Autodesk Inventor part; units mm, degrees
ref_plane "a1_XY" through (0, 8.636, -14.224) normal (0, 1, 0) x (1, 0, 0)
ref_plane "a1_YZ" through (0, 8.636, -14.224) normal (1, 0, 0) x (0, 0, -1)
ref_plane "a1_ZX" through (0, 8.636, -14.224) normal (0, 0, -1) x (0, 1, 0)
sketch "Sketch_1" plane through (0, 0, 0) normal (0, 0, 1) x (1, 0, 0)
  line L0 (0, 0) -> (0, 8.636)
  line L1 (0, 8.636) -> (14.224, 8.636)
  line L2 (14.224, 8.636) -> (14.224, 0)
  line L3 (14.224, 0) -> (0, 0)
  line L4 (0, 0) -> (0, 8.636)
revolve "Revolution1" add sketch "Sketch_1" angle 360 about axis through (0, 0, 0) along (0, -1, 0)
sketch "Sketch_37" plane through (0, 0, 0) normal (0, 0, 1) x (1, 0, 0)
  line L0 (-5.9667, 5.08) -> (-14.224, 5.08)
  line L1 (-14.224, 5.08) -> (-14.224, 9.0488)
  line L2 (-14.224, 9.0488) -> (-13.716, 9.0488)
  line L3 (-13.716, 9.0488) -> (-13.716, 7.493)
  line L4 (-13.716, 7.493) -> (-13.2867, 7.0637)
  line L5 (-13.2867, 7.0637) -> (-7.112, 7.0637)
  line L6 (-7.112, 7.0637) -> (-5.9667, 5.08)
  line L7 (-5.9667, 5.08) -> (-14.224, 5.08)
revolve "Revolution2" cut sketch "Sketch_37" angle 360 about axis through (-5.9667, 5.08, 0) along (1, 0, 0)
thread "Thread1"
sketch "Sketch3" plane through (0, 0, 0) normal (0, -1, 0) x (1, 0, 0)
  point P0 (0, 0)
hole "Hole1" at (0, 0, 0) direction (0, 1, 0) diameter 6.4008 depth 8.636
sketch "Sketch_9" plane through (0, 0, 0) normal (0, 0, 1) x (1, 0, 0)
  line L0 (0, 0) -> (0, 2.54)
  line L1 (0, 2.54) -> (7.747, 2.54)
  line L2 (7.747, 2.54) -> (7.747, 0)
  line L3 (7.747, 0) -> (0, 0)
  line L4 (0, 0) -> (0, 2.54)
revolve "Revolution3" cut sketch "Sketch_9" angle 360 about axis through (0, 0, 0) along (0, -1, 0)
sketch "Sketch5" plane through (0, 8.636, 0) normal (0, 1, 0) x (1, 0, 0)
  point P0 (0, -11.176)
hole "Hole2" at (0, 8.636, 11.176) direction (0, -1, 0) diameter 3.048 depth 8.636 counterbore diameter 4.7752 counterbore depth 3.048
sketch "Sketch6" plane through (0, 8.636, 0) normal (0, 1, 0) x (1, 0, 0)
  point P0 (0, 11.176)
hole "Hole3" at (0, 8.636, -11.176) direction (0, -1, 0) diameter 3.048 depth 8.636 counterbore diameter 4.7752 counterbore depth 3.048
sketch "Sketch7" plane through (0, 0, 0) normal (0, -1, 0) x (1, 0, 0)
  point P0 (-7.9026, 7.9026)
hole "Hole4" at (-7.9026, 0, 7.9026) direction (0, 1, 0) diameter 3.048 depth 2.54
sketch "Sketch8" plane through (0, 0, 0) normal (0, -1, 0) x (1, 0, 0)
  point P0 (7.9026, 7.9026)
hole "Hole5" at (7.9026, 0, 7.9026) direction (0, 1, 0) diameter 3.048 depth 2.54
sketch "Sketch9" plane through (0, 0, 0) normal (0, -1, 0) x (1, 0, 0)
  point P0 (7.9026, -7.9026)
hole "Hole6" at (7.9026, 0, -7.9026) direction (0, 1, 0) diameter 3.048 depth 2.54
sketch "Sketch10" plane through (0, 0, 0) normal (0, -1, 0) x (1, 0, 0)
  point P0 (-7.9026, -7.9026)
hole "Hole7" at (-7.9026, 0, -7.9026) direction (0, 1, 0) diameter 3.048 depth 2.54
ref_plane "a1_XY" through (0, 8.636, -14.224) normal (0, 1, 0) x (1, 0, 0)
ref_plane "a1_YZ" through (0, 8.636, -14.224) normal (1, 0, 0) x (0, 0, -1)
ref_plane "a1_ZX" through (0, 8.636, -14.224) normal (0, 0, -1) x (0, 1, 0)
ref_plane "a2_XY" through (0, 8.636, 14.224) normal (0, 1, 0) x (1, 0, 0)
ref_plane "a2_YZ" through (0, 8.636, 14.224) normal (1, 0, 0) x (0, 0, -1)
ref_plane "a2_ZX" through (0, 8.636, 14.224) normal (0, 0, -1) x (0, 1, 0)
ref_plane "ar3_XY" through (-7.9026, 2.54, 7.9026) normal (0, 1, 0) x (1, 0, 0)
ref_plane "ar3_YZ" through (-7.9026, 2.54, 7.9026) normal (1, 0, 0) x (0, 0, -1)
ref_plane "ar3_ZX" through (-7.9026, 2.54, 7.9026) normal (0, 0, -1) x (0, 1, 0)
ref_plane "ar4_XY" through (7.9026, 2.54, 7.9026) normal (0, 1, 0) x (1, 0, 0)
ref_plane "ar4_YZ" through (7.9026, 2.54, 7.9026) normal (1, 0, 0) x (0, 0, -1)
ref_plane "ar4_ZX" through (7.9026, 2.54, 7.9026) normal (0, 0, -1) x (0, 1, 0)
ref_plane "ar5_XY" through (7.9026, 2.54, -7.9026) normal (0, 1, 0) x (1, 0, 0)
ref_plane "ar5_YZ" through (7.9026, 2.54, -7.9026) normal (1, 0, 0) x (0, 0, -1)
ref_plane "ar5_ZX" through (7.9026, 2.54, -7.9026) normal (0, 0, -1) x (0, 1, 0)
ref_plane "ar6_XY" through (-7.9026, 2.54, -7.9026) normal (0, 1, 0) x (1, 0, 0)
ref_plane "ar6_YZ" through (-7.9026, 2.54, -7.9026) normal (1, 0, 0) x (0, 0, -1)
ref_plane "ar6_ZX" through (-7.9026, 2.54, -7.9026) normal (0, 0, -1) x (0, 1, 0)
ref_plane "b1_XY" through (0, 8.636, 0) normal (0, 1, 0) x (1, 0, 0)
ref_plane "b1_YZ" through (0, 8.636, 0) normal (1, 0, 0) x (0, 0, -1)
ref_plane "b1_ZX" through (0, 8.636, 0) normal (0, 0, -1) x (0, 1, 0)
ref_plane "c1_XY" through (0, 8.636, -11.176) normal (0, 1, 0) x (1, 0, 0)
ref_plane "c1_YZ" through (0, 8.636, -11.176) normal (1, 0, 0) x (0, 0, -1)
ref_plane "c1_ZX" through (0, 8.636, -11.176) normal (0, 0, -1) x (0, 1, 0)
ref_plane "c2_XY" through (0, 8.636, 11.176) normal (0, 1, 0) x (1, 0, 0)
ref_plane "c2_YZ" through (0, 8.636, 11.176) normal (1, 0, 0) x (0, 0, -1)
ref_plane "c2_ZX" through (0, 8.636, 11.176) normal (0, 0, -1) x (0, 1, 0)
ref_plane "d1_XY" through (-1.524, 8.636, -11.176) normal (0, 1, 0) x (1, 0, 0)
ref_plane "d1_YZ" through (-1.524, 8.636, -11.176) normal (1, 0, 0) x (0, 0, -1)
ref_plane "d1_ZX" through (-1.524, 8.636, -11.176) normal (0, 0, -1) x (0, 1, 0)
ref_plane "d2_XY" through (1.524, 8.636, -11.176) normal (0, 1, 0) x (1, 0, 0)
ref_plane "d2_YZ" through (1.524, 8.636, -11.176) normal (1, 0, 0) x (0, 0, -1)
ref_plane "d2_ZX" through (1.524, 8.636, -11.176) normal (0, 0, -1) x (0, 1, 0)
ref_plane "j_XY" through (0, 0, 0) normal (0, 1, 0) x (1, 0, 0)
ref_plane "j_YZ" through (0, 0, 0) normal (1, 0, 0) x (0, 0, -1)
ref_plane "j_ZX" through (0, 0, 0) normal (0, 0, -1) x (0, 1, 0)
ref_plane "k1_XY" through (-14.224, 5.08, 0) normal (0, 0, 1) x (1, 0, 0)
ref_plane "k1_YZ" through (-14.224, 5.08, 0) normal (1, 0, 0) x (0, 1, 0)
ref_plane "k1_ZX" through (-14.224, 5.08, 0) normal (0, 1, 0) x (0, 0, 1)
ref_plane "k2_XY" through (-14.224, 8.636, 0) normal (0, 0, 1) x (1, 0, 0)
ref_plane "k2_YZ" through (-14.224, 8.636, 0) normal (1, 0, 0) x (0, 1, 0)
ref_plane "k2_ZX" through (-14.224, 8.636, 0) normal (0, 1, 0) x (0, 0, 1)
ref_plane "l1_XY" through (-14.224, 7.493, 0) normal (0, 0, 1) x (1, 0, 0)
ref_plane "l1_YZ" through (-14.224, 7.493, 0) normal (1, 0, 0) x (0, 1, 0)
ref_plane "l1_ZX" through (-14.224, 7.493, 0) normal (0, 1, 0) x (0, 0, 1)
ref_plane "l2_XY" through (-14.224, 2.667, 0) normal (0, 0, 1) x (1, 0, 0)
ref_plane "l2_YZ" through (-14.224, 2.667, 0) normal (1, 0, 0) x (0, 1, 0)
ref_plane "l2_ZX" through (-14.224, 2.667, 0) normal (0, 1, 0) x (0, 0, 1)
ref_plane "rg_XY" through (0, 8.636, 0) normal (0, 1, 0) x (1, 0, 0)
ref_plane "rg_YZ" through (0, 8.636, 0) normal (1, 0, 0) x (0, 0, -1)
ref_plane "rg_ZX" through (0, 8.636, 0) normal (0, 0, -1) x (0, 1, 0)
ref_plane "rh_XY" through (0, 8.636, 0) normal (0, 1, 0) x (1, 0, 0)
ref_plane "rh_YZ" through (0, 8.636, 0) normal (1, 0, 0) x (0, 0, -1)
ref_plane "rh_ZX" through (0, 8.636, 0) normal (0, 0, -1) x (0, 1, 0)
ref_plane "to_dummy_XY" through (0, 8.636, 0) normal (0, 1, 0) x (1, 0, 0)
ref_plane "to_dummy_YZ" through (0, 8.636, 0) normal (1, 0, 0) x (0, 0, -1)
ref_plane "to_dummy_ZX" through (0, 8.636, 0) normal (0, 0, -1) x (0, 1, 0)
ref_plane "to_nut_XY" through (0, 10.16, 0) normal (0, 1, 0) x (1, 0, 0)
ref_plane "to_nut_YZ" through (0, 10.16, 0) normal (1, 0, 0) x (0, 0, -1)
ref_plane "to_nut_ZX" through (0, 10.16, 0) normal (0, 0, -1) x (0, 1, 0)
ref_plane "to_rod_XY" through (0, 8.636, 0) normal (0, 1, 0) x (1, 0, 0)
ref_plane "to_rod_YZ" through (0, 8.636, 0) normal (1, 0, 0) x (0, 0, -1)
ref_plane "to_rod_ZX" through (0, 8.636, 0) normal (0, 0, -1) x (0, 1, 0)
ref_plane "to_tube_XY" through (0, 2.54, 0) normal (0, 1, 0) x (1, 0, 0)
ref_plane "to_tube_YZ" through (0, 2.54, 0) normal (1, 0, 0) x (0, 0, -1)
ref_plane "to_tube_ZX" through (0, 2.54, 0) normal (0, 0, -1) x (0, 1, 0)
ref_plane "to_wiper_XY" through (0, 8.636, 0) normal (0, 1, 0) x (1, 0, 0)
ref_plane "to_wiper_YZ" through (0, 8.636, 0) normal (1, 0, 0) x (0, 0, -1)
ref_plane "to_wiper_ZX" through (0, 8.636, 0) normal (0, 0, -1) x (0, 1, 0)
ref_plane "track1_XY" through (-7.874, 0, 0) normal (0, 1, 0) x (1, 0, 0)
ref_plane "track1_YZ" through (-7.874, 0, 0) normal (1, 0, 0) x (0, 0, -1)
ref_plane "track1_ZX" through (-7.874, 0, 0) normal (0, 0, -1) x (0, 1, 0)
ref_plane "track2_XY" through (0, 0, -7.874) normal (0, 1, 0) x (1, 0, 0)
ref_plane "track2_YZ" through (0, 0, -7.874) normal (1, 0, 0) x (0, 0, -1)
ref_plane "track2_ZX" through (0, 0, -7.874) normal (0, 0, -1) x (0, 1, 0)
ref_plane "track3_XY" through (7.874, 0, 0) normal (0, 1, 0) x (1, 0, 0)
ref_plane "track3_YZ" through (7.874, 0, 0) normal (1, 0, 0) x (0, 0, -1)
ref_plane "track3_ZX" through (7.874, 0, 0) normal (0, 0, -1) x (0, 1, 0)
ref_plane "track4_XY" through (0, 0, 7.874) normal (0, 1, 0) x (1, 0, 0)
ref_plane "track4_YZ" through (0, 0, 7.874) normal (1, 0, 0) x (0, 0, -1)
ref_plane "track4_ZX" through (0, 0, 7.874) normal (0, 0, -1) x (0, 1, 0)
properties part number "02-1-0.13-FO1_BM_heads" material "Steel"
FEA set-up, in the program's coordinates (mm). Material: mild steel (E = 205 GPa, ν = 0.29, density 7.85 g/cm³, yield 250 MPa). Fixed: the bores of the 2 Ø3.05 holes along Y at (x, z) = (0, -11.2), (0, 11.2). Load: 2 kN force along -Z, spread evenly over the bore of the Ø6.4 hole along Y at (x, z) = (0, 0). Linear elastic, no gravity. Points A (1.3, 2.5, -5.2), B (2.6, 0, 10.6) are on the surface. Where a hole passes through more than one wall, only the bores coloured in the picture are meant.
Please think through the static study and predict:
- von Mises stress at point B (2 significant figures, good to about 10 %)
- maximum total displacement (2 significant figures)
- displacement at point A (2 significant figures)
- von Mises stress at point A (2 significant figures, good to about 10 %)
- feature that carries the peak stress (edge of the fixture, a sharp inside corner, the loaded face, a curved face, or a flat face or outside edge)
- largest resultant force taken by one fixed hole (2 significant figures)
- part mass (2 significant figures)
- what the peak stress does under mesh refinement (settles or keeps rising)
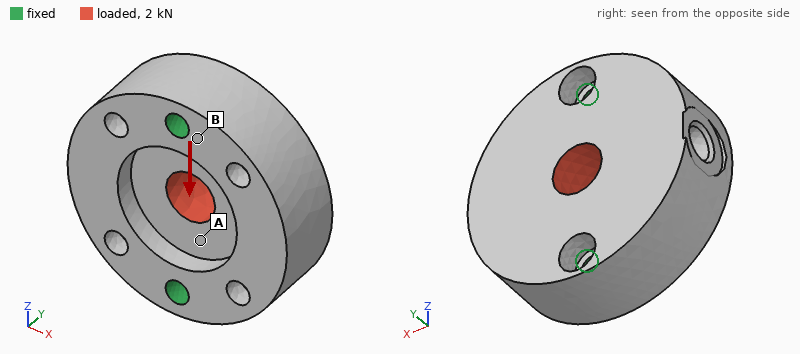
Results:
10 MPa
1.1 µm
0.64 µm
25 MPa
edge of the fixture
1.0 kN
35 g
keeps rising
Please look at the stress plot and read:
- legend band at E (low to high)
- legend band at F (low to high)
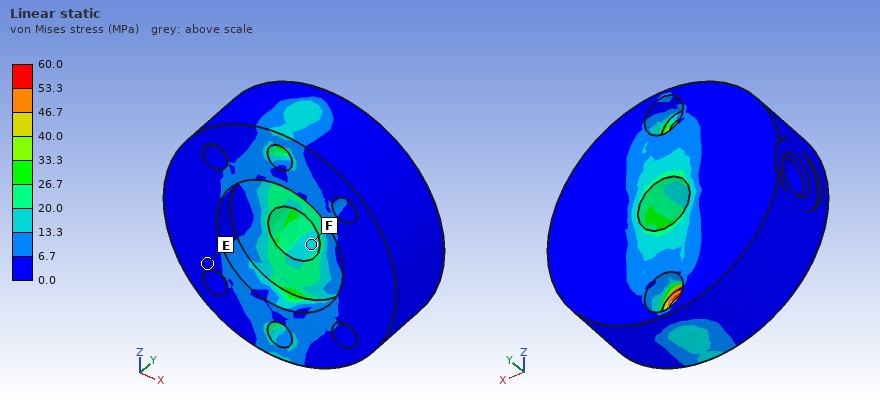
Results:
0.0 to 6.7 MPa
13.3 to 20.0 MPa
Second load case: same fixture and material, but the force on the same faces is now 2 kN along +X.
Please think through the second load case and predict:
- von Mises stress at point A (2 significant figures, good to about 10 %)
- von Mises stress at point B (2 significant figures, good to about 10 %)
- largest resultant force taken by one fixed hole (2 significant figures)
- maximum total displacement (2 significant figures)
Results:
15 MPa
16 MPa
1.0 kN
3.4 µm
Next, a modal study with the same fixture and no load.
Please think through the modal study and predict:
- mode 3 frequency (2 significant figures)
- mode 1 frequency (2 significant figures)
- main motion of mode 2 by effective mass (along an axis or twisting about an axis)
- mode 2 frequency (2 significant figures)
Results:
41 kHz
17 kHz
along Y
25 kHz
